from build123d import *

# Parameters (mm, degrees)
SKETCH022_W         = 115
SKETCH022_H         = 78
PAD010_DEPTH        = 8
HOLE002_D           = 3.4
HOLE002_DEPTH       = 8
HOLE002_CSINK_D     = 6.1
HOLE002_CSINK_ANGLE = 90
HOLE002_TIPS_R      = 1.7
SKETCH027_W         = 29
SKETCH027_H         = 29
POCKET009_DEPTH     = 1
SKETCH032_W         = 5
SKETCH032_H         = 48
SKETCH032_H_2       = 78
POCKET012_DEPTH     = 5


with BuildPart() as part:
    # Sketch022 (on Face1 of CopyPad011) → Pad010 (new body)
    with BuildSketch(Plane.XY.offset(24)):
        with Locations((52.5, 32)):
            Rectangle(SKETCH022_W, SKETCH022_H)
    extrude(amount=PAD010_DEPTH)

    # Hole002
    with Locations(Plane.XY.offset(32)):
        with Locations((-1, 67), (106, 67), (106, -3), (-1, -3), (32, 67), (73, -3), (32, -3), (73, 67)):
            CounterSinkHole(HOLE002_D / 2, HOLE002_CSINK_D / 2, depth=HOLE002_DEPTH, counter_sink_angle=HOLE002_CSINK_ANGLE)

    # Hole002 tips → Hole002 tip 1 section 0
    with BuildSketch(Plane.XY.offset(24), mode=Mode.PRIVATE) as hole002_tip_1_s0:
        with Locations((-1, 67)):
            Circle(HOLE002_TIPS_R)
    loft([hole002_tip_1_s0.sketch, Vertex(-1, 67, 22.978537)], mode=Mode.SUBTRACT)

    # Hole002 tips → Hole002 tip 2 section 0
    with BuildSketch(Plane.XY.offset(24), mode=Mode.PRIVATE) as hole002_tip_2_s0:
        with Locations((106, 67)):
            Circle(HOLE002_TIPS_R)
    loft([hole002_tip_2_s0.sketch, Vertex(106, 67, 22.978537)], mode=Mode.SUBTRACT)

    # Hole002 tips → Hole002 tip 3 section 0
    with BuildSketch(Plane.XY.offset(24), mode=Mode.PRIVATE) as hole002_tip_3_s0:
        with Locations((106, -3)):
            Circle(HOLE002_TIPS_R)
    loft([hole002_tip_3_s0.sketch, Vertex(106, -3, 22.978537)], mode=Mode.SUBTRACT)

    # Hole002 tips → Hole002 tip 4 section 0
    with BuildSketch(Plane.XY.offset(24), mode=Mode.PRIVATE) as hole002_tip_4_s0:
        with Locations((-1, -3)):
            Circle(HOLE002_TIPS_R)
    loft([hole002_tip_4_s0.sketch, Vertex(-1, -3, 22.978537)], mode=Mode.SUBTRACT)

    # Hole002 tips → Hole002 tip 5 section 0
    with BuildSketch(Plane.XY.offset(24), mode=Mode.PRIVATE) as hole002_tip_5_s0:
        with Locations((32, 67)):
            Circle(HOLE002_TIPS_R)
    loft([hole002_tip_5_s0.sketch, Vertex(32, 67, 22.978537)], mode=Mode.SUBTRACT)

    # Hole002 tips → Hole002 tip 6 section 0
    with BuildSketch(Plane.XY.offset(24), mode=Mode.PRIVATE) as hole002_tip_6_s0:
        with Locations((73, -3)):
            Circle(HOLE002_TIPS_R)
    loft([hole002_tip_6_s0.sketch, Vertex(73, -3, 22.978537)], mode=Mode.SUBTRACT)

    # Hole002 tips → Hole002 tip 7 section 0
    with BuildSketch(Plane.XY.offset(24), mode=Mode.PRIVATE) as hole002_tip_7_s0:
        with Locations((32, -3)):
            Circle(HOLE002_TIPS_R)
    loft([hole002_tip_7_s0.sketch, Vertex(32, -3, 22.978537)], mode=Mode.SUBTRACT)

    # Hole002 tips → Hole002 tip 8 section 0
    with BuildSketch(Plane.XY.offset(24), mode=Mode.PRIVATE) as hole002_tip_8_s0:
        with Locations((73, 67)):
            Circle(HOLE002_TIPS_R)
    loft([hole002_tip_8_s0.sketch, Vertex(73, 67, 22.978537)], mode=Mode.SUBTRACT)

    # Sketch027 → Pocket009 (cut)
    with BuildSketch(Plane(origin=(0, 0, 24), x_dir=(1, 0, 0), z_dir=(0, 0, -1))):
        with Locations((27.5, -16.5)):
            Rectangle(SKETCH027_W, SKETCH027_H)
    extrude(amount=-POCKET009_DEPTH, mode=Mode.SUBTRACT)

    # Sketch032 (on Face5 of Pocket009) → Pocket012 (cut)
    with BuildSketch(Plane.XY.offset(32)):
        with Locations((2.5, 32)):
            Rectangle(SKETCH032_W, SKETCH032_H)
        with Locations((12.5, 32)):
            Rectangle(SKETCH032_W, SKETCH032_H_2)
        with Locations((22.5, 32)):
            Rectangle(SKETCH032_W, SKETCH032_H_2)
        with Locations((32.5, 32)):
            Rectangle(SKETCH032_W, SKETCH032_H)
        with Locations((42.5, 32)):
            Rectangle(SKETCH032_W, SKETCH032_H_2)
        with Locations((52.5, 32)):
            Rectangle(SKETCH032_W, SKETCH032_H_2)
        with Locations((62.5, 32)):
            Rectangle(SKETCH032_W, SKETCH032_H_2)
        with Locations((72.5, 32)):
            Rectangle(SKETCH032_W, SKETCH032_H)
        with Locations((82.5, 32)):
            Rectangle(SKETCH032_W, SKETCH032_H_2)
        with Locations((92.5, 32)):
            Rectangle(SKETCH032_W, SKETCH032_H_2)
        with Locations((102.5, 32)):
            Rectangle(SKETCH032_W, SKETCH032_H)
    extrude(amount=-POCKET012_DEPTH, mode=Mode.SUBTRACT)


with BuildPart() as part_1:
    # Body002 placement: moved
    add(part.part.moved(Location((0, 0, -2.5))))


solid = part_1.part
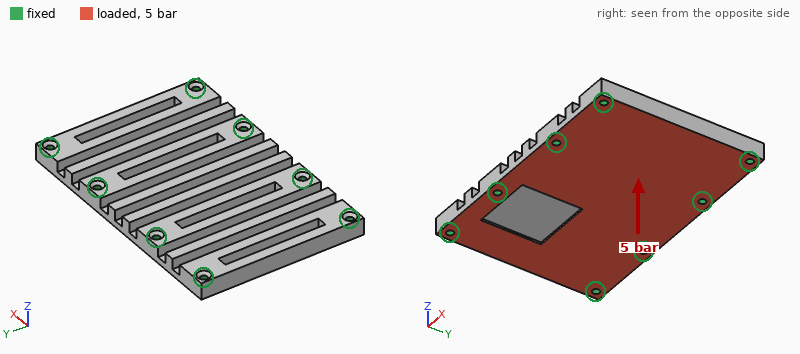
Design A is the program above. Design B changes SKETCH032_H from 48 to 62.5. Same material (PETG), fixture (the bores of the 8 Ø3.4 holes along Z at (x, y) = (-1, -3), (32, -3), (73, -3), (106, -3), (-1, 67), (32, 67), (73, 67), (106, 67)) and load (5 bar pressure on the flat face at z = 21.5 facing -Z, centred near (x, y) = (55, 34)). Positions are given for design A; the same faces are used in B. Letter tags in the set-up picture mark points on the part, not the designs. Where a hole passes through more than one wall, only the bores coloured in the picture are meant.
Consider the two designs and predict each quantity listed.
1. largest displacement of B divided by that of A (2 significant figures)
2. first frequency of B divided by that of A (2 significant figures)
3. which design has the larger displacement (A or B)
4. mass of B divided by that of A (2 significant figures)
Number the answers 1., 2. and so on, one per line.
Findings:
1. 1.1
2. 0.93
3. B
4. 0.97
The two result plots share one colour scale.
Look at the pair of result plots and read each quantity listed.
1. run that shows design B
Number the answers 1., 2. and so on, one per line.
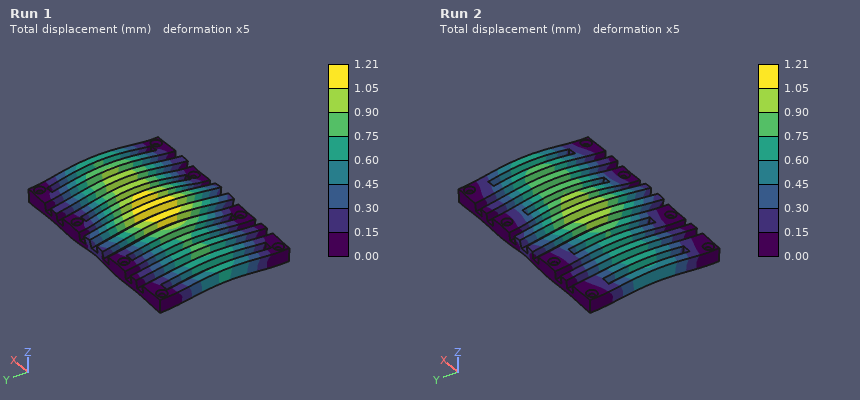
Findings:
1. Run 1
